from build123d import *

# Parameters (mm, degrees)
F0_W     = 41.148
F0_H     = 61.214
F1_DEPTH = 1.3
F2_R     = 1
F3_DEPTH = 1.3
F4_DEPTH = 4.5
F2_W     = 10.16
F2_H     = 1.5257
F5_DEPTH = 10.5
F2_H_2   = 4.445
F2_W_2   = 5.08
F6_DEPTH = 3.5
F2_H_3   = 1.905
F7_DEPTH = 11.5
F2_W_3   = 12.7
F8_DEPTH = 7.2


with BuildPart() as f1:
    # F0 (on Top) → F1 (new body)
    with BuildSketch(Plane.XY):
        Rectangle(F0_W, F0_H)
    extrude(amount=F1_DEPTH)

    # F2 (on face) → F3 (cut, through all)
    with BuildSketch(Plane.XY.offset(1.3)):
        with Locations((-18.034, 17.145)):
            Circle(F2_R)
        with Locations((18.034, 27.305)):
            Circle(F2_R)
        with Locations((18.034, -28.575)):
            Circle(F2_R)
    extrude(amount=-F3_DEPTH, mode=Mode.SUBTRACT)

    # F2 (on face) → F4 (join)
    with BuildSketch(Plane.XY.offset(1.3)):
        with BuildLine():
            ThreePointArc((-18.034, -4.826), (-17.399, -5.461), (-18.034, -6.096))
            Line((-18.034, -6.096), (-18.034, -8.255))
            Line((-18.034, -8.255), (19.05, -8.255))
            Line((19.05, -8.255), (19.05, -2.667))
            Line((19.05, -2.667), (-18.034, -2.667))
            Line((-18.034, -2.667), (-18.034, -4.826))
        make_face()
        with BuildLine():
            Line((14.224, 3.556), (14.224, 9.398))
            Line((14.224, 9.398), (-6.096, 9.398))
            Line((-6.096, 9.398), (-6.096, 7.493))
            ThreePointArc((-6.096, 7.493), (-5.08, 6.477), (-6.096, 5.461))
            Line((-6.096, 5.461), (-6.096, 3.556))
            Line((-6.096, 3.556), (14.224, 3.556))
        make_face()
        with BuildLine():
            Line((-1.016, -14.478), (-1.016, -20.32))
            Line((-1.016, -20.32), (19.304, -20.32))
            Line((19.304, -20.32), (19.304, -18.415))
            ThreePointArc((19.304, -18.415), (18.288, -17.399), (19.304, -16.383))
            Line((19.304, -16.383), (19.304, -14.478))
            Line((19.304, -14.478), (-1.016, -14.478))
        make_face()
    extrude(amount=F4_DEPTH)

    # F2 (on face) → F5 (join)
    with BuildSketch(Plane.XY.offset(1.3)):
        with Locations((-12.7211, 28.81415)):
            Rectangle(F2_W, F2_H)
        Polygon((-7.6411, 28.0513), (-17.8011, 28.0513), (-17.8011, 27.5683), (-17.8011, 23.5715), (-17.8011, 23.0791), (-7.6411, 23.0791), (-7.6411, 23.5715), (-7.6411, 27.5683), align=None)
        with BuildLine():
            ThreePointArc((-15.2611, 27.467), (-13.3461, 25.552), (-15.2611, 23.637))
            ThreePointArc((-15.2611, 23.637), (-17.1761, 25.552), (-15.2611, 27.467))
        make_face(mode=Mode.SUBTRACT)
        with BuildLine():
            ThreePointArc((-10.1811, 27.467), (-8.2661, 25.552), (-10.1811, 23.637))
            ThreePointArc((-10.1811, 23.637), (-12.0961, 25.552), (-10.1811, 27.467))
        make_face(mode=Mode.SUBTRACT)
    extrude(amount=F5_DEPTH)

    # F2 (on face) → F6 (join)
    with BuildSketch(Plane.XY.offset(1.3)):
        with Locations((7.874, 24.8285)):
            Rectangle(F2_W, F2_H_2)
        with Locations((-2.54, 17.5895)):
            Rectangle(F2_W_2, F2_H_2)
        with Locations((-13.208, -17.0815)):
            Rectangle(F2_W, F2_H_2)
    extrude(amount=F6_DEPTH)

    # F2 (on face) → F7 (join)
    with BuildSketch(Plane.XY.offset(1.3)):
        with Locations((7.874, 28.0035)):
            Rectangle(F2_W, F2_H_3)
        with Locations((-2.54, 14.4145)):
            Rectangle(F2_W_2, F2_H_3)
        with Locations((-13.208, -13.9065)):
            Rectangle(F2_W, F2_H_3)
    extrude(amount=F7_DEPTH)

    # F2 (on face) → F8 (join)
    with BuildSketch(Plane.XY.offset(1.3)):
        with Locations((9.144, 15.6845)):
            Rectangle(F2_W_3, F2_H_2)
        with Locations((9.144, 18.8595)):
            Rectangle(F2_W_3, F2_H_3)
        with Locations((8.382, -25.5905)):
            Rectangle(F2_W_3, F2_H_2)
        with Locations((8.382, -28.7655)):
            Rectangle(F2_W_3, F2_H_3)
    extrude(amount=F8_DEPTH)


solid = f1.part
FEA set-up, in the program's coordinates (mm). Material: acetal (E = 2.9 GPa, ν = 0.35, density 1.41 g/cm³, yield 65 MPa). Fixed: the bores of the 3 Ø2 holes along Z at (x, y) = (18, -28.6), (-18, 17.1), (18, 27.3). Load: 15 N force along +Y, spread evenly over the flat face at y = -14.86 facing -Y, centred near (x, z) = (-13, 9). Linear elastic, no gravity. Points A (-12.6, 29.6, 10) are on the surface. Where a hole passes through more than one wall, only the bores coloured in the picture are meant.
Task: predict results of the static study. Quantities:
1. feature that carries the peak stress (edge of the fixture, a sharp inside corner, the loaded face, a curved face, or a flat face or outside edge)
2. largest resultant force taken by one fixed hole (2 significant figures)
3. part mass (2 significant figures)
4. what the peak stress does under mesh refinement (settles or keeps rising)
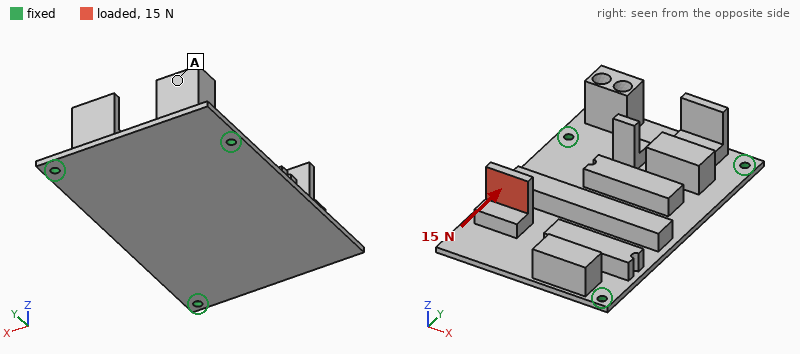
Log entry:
edge of the fixture
7.3 N
11 g
keeps rising
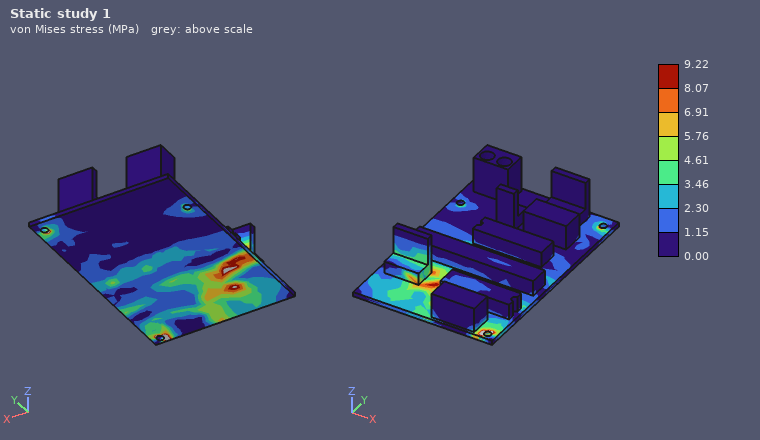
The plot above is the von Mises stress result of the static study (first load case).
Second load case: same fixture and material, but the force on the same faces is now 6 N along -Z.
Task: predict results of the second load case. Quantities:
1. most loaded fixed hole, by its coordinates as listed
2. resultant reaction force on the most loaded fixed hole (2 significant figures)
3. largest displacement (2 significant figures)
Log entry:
(-18, 17.1)
6.8 N
0.75 mm
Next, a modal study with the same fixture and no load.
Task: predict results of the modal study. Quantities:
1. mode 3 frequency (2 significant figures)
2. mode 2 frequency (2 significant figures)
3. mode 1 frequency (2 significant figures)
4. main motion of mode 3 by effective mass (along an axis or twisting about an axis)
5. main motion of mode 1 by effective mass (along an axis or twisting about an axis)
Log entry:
860 Hz
510 Hz
350 Hz
along Z
along Z
